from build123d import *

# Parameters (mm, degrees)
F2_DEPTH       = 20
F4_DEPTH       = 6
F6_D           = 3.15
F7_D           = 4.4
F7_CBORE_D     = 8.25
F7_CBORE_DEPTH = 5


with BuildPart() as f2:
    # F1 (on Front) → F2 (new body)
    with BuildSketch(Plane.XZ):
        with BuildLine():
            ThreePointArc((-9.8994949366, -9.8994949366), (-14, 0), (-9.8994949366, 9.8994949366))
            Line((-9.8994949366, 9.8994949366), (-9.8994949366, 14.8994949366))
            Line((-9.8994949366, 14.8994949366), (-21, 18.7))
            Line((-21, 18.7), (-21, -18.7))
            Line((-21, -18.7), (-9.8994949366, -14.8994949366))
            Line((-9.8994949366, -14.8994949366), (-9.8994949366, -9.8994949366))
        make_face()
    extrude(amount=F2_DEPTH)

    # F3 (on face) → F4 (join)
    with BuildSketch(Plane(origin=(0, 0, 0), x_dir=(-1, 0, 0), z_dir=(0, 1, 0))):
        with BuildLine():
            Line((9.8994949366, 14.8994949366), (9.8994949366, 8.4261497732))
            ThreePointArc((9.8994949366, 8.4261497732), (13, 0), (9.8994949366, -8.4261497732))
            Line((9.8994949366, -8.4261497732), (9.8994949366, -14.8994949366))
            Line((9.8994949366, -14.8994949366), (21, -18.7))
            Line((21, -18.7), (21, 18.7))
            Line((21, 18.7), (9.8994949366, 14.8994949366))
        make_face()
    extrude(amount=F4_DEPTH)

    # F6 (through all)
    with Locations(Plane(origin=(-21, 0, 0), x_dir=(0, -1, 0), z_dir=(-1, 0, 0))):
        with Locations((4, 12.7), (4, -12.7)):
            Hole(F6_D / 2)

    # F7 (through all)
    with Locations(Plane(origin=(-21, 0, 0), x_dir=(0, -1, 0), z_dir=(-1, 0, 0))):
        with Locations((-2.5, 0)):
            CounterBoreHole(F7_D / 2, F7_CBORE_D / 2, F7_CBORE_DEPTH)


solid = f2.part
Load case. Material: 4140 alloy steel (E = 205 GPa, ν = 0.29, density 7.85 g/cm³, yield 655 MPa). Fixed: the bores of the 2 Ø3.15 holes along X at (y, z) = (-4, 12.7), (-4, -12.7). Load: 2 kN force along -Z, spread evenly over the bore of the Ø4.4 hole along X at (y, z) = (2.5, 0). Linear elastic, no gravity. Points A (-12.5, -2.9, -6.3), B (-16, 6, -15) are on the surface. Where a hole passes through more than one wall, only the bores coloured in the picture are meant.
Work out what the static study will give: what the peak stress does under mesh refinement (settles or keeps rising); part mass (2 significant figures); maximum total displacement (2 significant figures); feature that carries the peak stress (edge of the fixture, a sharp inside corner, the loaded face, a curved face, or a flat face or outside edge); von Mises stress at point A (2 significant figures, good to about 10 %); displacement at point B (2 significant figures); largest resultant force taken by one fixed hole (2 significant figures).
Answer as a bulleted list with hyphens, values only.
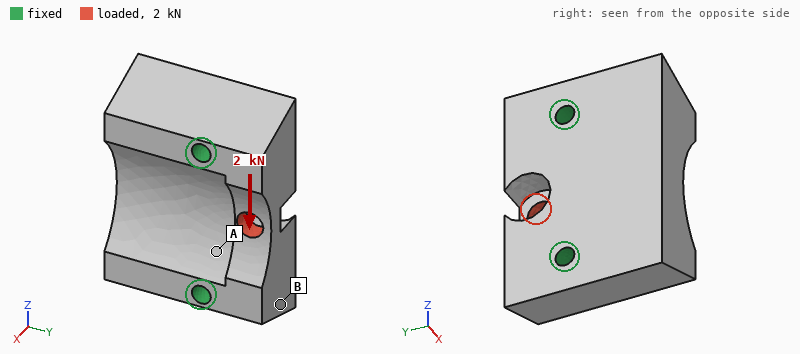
- keeps rising
- 62 g
- 2.5 µm
- a sharp inside corner
- 16 MPa
- 0.95 µm
- 1.1 kN
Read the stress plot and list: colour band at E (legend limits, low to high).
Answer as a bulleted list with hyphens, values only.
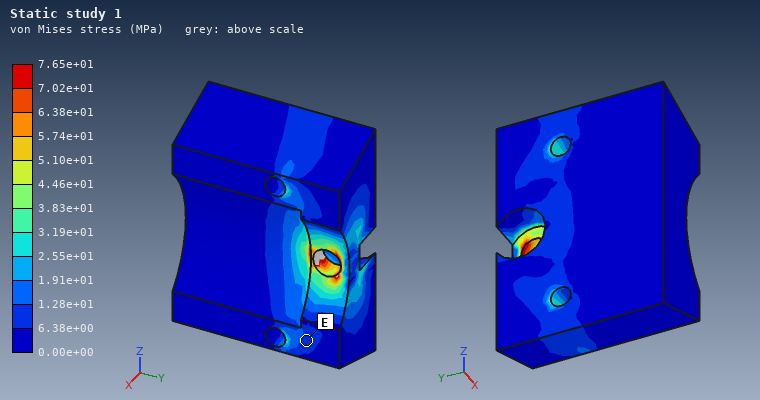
- 6.38e+00 to 1.28e+01 MPa
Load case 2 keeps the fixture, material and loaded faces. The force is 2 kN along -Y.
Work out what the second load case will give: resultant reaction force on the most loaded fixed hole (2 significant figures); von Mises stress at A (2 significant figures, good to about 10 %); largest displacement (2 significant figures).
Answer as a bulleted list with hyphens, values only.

- 1.0 kN
- 28 MPa
- 6.6 µm
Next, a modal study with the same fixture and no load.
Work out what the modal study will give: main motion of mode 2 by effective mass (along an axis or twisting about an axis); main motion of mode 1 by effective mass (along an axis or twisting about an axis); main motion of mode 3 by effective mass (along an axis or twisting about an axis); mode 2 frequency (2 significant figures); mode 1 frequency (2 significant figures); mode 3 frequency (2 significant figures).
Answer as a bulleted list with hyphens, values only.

- twisting about Y
- along X
- along Z
- 31 kHz
- 23 kHz
- 39 kHz
